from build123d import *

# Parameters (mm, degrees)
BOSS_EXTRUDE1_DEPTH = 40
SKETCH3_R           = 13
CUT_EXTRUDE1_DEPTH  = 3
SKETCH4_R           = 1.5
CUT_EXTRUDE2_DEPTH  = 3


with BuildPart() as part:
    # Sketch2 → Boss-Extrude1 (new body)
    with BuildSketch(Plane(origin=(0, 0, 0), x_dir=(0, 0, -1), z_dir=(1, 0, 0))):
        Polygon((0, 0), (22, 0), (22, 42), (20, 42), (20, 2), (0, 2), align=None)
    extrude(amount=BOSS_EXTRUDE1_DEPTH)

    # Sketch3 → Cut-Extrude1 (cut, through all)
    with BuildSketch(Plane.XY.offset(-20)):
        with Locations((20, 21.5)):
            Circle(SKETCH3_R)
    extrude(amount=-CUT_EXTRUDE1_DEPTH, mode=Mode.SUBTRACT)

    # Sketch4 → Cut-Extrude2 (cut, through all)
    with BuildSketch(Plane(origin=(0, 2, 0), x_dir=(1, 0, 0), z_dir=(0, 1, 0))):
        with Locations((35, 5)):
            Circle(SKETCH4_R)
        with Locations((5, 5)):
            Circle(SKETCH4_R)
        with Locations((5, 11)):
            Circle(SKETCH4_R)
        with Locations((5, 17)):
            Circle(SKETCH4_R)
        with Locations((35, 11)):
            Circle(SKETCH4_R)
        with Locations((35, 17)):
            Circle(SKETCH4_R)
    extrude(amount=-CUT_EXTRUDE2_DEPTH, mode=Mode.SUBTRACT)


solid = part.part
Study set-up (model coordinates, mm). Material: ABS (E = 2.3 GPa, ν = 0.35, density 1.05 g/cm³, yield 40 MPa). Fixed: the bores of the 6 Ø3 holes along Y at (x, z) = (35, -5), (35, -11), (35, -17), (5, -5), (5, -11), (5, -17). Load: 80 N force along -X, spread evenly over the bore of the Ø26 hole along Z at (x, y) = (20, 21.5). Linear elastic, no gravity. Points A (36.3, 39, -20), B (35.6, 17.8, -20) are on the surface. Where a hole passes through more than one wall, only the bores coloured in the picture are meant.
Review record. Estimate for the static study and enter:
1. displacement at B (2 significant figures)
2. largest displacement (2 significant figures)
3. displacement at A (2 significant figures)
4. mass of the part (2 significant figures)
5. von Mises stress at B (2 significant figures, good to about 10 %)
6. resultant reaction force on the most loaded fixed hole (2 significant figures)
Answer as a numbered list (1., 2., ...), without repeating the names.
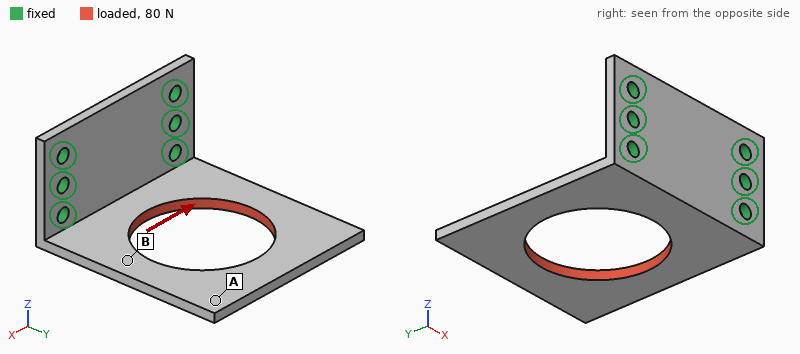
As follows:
1. 0.21 mm
2. 0.45 mm
3. 0.41 mm
4. 4.0 g
5. 4.7 MPa
6. 63 N
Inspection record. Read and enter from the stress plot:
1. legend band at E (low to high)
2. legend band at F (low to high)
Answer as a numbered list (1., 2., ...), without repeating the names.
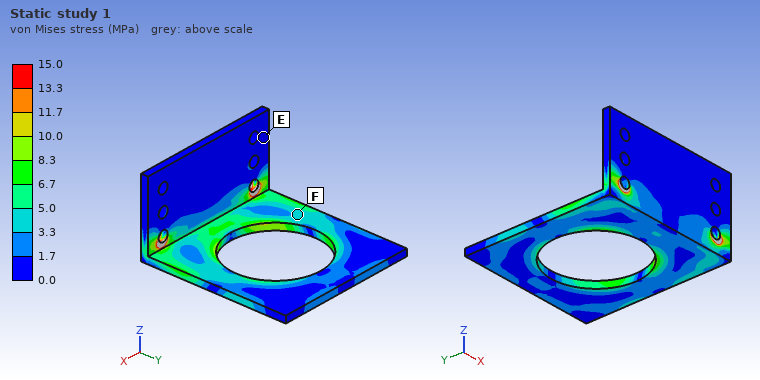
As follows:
1. 0.0 to 1.7 MPa
2. 3.3 to 5.0 MPa
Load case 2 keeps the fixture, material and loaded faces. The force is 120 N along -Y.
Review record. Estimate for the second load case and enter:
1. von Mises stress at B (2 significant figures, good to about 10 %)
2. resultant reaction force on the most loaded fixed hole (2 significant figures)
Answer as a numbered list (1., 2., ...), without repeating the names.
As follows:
1. 2.9 MPa
2. 67 N
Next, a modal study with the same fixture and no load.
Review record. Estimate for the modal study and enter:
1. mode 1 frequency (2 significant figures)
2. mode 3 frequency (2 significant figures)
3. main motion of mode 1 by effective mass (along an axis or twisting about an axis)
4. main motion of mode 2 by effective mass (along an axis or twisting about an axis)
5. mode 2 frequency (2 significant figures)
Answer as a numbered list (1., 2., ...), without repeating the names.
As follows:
1. 230 Hz
2. 1500 Hz
3. along Z
4. twisting about Y
5. 550 Hz
